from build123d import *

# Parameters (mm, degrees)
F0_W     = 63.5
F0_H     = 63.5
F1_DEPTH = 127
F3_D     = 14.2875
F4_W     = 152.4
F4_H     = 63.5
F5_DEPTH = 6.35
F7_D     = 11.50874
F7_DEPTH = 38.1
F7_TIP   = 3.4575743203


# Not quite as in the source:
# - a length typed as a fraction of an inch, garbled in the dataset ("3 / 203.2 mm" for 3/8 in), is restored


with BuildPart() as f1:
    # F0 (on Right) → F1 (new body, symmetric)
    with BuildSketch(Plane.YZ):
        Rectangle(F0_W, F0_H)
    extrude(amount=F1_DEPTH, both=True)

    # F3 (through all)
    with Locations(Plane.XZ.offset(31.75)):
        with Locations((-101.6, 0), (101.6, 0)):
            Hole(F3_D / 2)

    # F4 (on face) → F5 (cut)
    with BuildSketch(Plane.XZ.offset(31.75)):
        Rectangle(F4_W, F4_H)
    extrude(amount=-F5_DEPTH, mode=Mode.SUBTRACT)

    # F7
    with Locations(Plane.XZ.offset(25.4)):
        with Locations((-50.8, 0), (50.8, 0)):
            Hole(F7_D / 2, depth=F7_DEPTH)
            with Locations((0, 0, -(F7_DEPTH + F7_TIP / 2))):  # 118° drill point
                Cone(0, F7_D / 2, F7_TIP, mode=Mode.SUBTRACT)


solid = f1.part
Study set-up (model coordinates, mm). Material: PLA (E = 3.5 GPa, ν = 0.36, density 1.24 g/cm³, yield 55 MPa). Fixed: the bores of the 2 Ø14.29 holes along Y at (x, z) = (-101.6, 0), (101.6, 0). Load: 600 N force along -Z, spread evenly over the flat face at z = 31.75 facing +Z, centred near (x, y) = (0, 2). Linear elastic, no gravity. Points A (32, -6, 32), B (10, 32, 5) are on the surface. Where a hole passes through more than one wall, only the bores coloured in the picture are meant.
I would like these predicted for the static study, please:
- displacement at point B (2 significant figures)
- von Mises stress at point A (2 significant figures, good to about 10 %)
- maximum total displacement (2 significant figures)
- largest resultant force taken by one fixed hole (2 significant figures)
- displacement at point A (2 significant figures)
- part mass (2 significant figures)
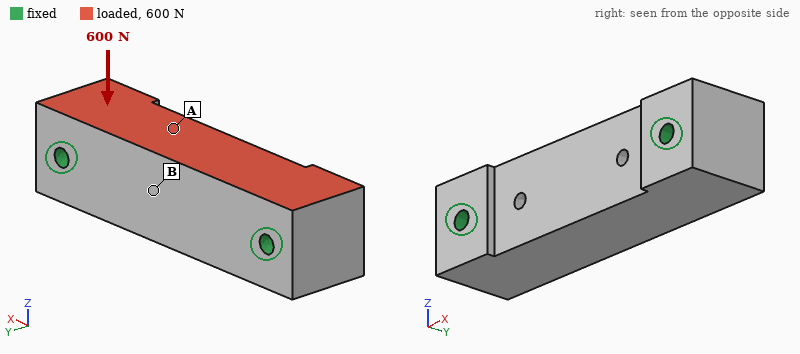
8.4 µm
0.15 MPa
8.5 µm
300 N
7.4 µm
1.2 kg
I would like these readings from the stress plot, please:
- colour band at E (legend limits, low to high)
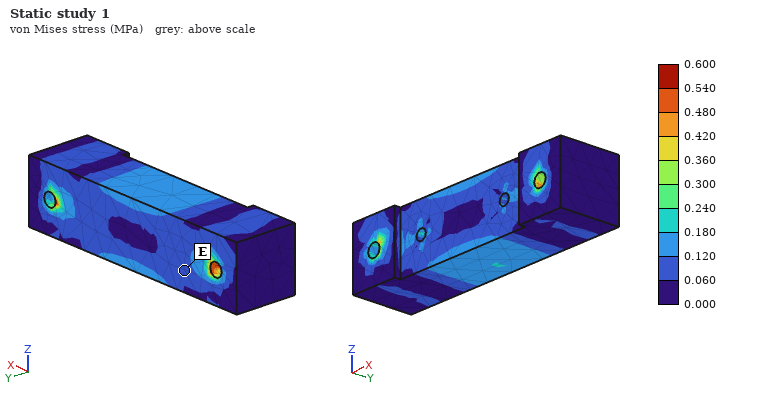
0.060 to 0.120 MPa
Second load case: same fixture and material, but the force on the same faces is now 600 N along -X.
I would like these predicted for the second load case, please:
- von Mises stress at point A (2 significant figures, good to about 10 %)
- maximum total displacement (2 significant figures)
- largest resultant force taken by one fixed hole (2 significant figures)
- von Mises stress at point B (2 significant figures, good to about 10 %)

0.071 MPa
2.6 µm
310 N
0.046 MPa
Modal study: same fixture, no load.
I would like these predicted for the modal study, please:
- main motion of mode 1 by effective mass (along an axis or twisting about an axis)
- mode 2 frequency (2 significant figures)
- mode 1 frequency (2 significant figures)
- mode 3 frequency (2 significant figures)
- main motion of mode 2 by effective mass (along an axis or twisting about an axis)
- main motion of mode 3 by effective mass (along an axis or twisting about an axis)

along Z
1700 Hz
1300 Hz
2300 Hz
along Y
twisting about X
